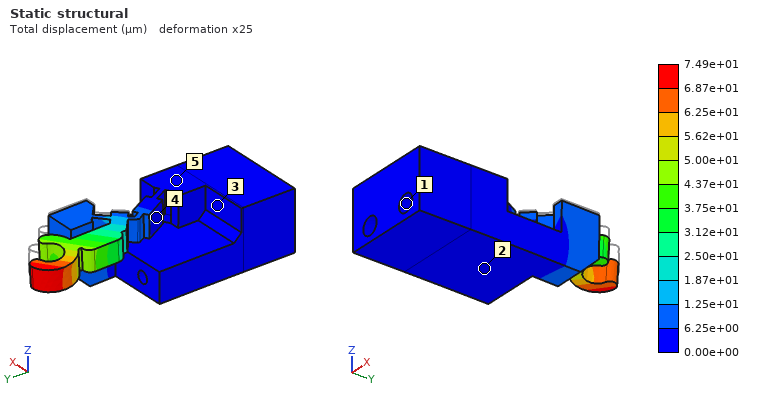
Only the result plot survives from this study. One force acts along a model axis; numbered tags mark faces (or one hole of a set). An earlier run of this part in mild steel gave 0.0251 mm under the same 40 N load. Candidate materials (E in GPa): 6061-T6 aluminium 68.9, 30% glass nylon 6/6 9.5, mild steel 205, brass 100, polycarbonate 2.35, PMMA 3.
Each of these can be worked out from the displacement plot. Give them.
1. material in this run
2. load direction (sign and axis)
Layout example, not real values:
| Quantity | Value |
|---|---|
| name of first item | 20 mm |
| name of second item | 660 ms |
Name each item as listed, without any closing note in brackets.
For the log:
| Quantity | Value |
|---|---|
| material in this run | 6061-T6 aluminium |
| load direction | -Z |
